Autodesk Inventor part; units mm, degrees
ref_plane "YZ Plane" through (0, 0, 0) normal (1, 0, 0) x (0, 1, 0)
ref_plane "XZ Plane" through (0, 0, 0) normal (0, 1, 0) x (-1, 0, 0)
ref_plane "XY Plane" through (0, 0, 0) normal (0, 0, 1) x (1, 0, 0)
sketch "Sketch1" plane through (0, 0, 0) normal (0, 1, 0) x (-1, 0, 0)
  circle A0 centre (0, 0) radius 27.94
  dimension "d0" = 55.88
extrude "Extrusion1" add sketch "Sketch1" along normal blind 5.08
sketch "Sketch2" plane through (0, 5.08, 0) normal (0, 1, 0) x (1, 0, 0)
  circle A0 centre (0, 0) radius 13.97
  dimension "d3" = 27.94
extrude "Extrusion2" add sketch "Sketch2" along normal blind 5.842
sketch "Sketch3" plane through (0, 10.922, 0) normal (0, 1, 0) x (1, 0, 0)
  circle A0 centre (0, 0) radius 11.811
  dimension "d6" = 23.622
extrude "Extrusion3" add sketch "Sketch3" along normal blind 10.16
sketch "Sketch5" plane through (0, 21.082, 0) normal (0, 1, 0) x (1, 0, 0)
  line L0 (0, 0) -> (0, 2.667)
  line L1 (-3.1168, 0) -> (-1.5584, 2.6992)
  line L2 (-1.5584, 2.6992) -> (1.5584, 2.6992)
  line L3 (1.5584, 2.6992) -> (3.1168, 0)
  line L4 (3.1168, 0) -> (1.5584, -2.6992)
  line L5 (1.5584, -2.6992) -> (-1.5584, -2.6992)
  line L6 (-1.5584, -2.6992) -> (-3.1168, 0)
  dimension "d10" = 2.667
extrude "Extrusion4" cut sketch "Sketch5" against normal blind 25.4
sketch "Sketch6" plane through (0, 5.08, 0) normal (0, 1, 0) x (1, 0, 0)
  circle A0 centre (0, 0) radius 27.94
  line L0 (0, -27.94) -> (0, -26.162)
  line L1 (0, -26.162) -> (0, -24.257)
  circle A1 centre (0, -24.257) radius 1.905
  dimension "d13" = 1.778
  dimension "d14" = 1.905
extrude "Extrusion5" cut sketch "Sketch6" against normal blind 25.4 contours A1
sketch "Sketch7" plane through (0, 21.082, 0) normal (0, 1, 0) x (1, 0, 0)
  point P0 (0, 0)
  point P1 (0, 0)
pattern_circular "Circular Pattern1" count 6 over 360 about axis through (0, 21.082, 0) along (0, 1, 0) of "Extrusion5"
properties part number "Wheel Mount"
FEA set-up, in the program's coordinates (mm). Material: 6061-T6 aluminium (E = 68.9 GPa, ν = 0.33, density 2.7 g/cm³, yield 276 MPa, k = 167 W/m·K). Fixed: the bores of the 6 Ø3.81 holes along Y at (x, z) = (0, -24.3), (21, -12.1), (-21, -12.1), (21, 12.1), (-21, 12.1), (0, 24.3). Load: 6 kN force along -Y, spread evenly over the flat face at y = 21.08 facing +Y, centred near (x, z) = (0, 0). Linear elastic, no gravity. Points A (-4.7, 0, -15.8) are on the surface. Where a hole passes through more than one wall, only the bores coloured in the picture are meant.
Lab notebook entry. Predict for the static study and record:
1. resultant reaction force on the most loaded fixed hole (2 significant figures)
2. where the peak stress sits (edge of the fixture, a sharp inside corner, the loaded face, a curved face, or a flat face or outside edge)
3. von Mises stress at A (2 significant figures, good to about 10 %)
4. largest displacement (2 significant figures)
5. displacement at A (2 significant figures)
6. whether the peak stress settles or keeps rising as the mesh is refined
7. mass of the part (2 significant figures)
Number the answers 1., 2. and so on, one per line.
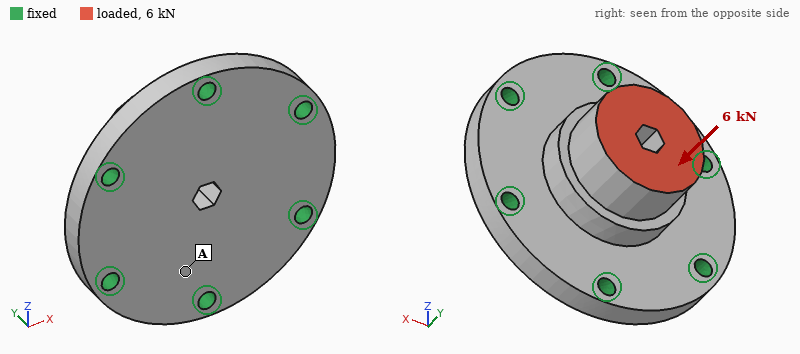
1. 1.1 kN
2. edge of the fixture
3. 24 MPa
4. 25 µm
5. 15 µm
6. keeps rising
7. 53 g
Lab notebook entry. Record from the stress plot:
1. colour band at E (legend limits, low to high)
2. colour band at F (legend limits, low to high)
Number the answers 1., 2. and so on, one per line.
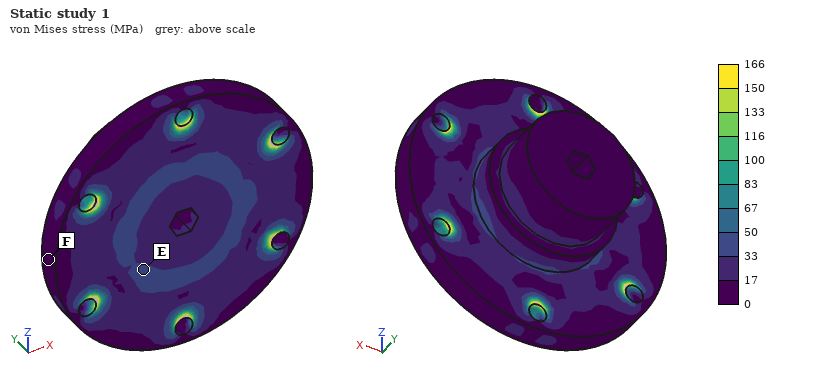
1. 33 to 50 MPa
2. 0 to 17 MPa
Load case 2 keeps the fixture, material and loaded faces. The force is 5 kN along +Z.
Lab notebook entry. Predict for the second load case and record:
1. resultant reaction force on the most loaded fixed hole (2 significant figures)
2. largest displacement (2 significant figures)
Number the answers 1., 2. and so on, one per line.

1. 2.0 kN
2. 51 µm
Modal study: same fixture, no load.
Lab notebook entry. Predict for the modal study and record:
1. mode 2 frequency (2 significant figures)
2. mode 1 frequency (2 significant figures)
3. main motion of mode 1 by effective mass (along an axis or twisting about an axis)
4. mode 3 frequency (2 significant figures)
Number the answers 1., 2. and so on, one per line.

1. 17 kHz
2. 14 kHz
3. along Y
4. 17 kHz
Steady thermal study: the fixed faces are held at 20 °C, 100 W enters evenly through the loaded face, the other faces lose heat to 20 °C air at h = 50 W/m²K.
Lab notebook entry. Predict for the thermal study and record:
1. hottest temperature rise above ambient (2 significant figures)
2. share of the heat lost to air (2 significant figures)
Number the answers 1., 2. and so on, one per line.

1. 38 K
2. 3.9 %
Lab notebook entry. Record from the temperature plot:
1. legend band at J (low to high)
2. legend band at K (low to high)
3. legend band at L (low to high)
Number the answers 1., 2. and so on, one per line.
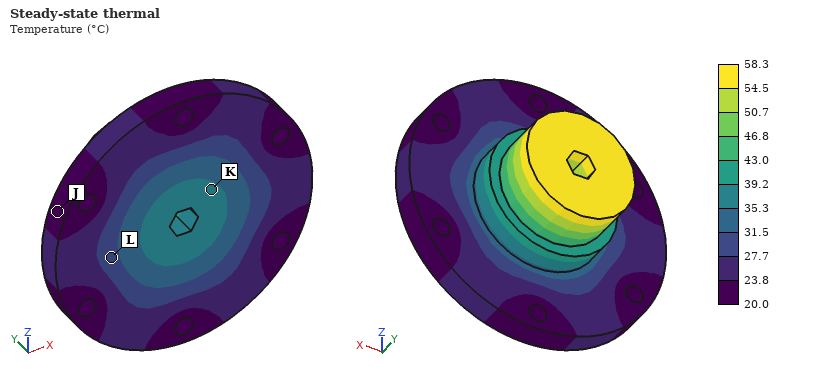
1. 20.0 to 23.8 °C
2. 35.3 to 39.2 °C
3. 27.7 to 31.5 °C
